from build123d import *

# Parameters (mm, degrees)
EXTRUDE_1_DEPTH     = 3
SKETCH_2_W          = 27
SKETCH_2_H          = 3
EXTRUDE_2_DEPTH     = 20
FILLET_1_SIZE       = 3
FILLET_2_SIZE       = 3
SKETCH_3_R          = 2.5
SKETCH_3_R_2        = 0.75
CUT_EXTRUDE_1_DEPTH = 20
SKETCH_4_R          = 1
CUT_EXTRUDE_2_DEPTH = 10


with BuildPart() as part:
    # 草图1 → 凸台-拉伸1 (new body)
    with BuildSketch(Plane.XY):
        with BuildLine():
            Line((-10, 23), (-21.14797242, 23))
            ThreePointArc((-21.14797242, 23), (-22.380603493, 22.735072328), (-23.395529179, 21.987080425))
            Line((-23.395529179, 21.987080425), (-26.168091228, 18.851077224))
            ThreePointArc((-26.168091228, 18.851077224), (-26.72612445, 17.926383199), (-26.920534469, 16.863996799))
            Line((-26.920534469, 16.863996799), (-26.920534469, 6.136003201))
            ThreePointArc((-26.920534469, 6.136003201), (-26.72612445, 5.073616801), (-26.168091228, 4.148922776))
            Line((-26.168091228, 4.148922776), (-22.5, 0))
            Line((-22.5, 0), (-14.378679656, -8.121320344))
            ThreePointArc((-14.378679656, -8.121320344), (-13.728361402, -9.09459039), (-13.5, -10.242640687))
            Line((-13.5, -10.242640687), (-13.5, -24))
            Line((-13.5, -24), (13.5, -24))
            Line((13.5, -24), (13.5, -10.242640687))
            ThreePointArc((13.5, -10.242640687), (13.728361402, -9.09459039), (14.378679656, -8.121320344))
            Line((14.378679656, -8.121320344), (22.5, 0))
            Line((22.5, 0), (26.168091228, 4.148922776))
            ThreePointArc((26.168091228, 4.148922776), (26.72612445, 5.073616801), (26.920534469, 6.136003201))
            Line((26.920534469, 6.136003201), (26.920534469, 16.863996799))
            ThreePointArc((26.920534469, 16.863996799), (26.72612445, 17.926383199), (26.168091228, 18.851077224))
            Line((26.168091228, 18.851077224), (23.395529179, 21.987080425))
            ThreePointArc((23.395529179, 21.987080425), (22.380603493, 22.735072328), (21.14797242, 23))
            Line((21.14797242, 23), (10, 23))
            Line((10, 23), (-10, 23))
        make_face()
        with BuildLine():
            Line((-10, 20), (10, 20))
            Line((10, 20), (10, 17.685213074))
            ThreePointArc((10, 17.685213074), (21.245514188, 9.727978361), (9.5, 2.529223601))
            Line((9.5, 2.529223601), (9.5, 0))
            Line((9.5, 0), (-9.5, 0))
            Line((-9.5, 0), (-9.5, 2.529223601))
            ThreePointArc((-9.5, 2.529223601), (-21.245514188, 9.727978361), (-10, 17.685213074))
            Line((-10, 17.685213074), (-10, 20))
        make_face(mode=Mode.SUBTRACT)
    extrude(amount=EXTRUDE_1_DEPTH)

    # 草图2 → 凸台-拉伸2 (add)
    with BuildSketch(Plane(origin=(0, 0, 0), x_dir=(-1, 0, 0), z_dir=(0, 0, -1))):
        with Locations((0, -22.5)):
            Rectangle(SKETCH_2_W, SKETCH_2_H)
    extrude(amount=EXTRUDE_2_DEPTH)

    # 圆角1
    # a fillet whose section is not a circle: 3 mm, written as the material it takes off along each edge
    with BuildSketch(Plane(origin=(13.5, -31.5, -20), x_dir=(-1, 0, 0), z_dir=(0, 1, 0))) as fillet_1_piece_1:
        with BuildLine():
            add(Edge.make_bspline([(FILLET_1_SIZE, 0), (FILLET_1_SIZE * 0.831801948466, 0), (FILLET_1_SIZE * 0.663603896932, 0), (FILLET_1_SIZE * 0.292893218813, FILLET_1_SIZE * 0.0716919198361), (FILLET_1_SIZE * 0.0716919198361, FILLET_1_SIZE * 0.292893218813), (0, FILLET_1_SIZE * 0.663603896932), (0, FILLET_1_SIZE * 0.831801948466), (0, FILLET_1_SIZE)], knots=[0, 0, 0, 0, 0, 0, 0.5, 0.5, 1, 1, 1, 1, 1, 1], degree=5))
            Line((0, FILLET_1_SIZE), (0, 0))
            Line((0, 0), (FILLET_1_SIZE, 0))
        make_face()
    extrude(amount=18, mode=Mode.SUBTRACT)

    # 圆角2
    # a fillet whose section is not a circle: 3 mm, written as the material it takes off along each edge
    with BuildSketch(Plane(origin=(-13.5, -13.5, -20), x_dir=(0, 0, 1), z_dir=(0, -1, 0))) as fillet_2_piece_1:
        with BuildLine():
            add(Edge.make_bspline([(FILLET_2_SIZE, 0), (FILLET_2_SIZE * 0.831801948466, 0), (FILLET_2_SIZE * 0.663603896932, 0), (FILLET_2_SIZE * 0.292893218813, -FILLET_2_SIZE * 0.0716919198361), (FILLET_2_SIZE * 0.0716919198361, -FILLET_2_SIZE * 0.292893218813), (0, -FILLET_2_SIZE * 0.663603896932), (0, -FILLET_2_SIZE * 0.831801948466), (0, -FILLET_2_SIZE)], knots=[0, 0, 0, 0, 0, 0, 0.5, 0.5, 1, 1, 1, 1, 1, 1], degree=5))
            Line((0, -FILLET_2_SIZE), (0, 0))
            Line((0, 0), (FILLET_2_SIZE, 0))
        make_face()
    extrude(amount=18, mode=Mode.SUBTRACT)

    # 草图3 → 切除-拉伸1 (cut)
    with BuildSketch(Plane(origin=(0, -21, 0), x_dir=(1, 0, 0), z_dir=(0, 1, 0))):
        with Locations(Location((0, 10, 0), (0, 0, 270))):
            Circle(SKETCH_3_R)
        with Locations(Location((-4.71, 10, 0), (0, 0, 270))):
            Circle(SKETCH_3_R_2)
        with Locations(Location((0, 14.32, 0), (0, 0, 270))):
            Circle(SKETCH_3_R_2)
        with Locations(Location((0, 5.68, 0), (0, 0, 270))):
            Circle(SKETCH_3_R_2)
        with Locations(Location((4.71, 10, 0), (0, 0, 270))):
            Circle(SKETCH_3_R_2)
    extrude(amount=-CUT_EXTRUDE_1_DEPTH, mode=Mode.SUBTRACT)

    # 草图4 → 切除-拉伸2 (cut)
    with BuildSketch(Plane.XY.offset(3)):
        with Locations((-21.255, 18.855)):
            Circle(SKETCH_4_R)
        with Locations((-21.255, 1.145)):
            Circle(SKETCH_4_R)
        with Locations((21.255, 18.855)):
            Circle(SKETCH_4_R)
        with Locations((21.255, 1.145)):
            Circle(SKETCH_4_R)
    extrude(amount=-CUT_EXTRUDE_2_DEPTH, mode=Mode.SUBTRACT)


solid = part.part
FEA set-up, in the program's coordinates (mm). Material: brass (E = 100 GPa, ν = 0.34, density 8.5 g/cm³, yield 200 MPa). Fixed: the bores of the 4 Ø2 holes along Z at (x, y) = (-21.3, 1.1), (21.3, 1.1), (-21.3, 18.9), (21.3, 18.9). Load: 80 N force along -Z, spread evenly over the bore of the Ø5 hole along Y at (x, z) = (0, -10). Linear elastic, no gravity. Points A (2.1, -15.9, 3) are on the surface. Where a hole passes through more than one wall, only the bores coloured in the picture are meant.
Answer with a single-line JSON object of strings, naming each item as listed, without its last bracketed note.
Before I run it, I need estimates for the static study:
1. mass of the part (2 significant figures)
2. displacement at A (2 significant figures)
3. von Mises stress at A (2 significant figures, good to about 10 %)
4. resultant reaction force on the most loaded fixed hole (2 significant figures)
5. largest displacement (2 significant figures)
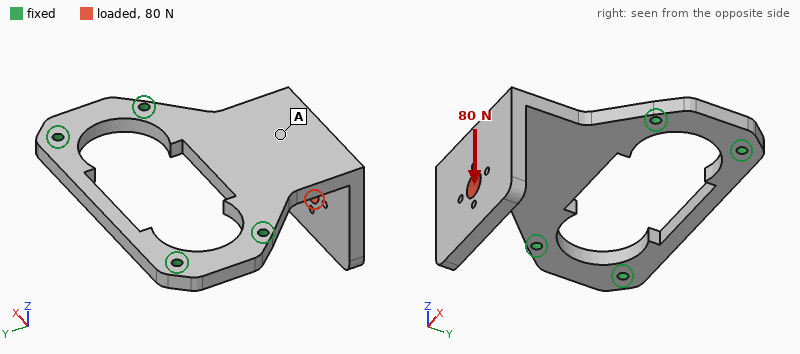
{"mass of the part": "44 g", "displacement at A": "0.10 mm", "von Mises stress at A": "14 MPa", "resultant reaction force on the most loaded fixed hole": "46 N", "largest displacement": "0.23 mm"}
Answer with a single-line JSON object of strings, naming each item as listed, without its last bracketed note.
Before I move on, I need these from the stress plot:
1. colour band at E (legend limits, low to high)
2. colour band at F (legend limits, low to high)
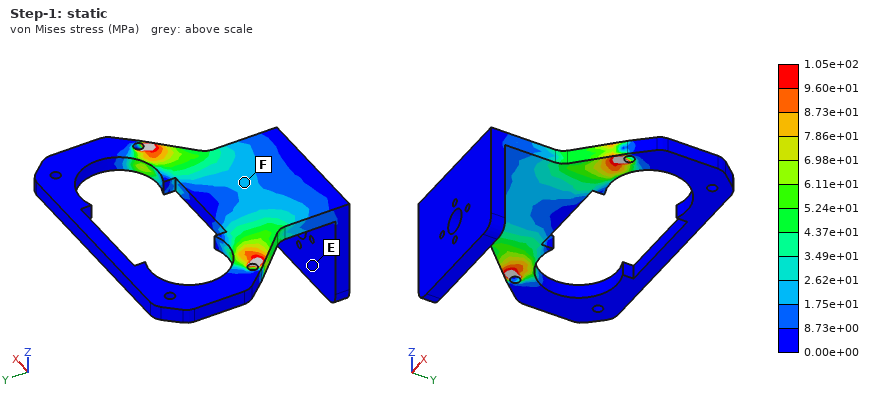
{"colour band at E": "0.00e+00 to 8.73e+00 MPa", "colour band at F": "1.75e+01 to 2.62e+01 MPa"}
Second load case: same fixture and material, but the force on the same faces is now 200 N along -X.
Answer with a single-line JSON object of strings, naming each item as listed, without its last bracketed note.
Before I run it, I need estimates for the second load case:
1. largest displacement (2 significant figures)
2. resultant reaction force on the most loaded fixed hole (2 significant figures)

{"largest displacement": "0.10 mm", "resultant reaction force on the most loaded fixed hole": "170 N"}
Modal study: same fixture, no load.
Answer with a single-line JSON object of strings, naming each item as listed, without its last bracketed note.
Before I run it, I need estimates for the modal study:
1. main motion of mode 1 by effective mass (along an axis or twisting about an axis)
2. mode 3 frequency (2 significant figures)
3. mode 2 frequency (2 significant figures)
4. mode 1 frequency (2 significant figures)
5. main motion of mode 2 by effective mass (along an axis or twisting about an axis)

{"main motion of mode 1 by effective mass": "along Z", "mode 3 frequency": "2600 Hz", "mode 2 frequency": "2000 Hz", "mode 1 frequency": "740 Hz", "main motion of mode 2 by effective mass": "along X"}
